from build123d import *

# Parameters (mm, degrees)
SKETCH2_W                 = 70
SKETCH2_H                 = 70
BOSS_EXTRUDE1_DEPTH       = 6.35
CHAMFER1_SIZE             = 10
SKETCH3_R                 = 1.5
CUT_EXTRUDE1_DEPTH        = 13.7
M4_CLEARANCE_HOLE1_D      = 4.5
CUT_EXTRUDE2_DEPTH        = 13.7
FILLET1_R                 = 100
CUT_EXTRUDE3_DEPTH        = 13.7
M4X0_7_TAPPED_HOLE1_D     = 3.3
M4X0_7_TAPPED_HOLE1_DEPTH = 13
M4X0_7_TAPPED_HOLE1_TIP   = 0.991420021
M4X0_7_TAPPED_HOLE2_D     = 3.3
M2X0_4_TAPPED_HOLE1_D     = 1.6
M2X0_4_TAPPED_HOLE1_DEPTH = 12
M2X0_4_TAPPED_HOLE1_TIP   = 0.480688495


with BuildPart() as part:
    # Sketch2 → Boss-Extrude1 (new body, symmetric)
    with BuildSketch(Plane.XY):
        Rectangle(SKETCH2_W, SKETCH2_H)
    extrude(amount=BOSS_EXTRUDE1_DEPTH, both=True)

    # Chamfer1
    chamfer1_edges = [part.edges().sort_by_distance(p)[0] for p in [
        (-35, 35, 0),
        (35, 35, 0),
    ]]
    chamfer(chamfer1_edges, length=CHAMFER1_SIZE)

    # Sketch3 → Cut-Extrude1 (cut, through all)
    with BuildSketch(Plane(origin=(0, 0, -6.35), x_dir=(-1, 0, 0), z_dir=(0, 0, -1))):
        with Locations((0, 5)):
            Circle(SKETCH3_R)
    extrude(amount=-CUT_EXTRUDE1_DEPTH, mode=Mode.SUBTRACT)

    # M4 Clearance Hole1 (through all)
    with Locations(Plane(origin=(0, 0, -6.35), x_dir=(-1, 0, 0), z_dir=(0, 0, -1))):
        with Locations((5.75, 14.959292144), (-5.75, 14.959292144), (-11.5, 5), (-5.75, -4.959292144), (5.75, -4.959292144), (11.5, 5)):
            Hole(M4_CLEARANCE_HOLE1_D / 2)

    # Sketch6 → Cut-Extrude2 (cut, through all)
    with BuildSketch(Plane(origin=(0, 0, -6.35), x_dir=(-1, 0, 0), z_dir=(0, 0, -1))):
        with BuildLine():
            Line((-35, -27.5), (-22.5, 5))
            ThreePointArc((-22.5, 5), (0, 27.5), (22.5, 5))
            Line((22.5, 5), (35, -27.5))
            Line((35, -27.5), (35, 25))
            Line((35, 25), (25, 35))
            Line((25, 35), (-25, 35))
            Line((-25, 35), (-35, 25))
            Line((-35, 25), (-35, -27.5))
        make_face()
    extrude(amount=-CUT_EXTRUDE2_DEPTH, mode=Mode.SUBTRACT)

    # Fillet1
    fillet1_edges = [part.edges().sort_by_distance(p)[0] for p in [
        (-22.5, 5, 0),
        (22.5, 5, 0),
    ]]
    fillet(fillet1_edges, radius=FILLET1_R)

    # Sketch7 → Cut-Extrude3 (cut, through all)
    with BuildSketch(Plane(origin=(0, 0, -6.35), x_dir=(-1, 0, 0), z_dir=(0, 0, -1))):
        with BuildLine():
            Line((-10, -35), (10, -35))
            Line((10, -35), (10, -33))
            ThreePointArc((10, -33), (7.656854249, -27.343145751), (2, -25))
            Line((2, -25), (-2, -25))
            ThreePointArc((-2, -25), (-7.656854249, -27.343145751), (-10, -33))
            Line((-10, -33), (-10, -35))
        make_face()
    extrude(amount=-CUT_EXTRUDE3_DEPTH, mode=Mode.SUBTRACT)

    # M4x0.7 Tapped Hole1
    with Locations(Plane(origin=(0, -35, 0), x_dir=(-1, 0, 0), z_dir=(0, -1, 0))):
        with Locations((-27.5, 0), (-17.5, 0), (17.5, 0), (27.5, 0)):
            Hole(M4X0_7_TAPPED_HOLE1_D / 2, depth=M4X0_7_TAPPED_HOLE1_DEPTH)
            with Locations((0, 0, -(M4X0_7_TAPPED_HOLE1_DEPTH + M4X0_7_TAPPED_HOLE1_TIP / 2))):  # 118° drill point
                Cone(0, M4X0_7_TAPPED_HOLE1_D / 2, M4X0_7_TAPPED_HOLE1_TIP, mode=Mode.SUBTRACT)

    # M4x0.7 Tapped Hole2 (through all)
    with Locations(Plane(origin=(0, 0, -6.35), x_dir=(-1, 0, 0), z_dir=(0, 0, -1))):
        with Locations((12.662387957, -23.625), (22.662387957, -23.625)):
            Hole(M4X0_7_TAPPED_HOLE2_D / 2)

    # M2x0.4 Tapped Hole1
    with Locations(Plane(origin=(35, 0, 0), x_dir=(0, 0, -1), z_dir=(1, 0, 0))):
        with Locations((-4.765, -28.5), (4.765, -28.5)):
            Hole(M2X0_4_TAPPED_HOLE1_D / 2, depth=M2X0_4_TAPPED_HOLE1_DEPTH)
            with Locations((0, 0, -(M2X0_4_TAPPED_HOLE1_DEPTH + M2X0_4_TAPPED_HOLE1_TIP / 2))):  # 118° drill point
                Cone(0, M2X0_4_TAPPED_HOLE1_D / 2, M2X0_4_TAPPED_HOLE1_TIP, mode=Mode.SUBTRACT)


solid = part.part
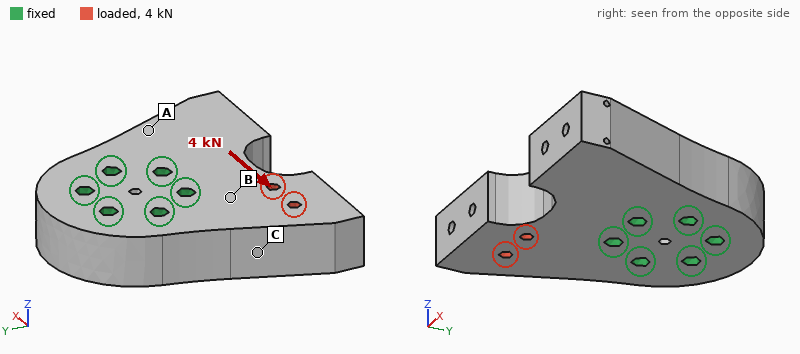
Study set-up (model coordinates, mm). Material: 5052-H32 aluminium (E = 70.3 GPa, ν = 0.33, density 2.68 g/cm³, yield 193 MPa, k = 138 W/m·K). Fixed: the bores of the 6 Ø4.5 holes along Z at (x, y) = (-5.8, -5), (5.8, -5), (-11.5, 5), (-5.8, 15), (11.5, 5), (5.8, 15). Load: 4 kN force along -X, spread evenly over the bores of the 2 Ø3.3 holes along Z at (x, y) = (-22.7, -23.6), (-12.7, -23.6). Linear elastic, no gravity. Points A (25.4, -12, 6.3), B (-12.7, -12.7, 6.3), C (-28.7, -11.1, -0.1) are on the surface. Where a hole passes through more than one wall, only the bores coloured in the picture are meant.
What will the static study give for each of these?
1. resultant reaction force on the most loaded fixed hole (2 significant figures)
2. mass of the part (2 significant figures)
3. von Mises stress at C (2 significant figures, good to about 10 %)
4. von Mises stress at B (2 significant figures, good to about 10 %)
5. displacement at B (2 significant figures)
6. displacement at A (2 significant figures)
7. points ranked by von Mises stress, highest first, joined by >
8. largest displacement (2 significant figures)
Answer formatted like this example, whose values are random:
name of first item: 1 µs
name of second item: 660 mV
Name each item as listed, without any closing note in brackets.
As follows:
resultant reaction force on the most loaded fixed hole: 2.7 kN
mass of the part: 97 g
von Mises stress at C: 9.7 MPa
von Mises stress at B: 16 MPa
displacement at B: 5.0 µm
displacement at A: 4.8 µm
points ranked by von Mises stress, highest first, joined by >: B > C > A
largest displacement: 22 µm
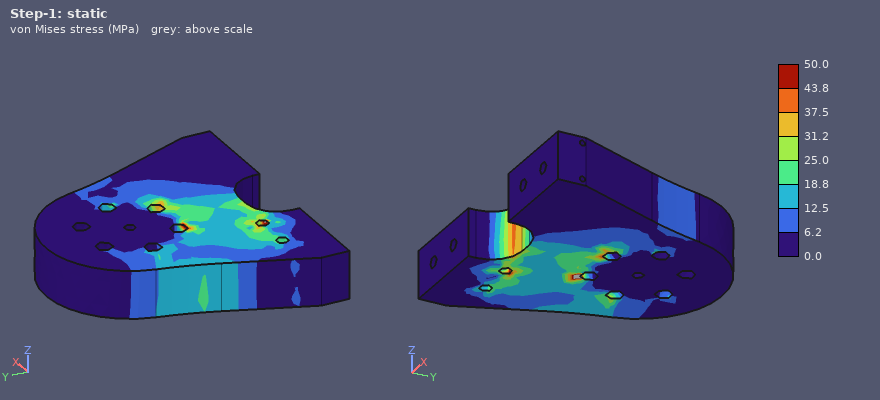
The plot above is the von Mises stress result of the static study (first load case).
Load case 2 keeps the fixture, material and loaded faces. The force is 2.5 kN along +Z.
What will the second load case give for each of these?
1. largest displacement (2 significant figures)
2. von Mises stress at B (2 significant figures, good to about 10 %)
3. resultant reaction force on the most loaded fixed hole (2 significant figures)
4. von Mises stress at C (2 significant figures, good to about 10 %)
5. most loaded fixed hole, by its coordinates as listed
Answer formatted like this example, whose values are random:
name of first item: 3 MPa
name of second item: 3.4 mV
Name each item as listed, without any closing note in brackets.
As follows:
largest displacement: 66 µm
von Mises stress at B: 36 MPa
resultant reaction force on the most loaded fixed hole: 2.4 kN
von Mises stress at C: 14 MPa
most loaded fixed hole, by its coordinates as listed: (-5.8, -5)
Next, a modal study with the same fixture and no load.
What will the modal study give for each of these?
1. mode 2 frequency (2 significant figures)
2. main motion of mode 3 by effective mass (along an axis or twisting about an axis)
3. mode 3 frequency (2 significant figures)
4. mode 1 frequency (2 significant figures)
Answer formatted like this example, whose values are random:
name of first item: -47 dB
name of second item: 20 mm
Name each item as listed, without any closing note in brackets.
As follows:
mode 2 frequency: 8300 Hz
main motion of mode 3 by effective mass: along X
mode 3 frequency: 13 kHz
mode 1 frequency: 8200 Hz
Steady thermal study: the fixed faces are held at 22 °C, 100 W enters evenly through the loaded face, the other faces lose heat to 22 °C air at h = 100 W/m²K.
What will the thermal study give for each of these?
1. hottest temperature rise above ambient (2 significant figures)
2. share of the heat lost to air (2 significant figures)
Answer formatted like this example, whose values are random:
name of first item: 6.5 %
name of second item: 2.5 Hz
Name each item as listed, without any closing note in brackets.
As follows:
hottest temperature rise above ambient: 46 K
share of the heat lost to air: 11 %
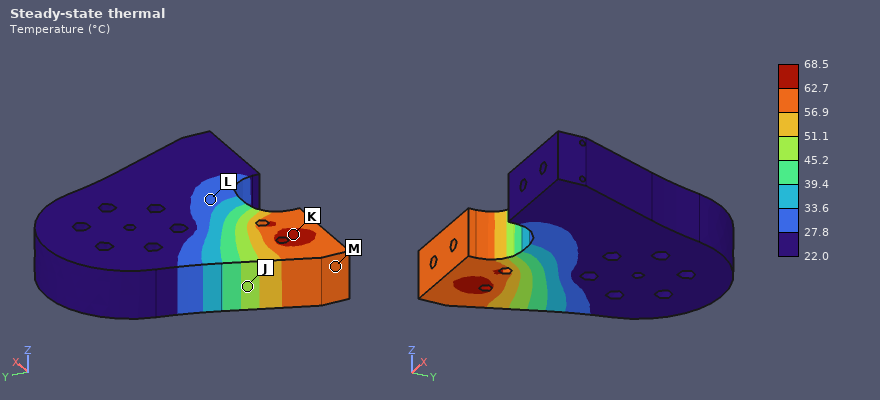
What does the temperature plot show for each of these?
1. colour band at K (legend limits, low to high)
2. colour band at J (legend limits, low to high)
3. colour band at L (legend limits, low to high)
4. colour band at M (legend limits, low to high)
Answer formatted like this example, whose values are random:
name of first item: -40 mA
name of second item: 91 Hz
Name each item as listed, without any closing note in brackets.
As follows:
colour band at K: 62.7 to 68.5 °C
colour band at J: 45.2 to 51.1 °C
colour band at L: 27.8 to 33.6 °C
colour band at M: 56.9 to 62.7 °C
